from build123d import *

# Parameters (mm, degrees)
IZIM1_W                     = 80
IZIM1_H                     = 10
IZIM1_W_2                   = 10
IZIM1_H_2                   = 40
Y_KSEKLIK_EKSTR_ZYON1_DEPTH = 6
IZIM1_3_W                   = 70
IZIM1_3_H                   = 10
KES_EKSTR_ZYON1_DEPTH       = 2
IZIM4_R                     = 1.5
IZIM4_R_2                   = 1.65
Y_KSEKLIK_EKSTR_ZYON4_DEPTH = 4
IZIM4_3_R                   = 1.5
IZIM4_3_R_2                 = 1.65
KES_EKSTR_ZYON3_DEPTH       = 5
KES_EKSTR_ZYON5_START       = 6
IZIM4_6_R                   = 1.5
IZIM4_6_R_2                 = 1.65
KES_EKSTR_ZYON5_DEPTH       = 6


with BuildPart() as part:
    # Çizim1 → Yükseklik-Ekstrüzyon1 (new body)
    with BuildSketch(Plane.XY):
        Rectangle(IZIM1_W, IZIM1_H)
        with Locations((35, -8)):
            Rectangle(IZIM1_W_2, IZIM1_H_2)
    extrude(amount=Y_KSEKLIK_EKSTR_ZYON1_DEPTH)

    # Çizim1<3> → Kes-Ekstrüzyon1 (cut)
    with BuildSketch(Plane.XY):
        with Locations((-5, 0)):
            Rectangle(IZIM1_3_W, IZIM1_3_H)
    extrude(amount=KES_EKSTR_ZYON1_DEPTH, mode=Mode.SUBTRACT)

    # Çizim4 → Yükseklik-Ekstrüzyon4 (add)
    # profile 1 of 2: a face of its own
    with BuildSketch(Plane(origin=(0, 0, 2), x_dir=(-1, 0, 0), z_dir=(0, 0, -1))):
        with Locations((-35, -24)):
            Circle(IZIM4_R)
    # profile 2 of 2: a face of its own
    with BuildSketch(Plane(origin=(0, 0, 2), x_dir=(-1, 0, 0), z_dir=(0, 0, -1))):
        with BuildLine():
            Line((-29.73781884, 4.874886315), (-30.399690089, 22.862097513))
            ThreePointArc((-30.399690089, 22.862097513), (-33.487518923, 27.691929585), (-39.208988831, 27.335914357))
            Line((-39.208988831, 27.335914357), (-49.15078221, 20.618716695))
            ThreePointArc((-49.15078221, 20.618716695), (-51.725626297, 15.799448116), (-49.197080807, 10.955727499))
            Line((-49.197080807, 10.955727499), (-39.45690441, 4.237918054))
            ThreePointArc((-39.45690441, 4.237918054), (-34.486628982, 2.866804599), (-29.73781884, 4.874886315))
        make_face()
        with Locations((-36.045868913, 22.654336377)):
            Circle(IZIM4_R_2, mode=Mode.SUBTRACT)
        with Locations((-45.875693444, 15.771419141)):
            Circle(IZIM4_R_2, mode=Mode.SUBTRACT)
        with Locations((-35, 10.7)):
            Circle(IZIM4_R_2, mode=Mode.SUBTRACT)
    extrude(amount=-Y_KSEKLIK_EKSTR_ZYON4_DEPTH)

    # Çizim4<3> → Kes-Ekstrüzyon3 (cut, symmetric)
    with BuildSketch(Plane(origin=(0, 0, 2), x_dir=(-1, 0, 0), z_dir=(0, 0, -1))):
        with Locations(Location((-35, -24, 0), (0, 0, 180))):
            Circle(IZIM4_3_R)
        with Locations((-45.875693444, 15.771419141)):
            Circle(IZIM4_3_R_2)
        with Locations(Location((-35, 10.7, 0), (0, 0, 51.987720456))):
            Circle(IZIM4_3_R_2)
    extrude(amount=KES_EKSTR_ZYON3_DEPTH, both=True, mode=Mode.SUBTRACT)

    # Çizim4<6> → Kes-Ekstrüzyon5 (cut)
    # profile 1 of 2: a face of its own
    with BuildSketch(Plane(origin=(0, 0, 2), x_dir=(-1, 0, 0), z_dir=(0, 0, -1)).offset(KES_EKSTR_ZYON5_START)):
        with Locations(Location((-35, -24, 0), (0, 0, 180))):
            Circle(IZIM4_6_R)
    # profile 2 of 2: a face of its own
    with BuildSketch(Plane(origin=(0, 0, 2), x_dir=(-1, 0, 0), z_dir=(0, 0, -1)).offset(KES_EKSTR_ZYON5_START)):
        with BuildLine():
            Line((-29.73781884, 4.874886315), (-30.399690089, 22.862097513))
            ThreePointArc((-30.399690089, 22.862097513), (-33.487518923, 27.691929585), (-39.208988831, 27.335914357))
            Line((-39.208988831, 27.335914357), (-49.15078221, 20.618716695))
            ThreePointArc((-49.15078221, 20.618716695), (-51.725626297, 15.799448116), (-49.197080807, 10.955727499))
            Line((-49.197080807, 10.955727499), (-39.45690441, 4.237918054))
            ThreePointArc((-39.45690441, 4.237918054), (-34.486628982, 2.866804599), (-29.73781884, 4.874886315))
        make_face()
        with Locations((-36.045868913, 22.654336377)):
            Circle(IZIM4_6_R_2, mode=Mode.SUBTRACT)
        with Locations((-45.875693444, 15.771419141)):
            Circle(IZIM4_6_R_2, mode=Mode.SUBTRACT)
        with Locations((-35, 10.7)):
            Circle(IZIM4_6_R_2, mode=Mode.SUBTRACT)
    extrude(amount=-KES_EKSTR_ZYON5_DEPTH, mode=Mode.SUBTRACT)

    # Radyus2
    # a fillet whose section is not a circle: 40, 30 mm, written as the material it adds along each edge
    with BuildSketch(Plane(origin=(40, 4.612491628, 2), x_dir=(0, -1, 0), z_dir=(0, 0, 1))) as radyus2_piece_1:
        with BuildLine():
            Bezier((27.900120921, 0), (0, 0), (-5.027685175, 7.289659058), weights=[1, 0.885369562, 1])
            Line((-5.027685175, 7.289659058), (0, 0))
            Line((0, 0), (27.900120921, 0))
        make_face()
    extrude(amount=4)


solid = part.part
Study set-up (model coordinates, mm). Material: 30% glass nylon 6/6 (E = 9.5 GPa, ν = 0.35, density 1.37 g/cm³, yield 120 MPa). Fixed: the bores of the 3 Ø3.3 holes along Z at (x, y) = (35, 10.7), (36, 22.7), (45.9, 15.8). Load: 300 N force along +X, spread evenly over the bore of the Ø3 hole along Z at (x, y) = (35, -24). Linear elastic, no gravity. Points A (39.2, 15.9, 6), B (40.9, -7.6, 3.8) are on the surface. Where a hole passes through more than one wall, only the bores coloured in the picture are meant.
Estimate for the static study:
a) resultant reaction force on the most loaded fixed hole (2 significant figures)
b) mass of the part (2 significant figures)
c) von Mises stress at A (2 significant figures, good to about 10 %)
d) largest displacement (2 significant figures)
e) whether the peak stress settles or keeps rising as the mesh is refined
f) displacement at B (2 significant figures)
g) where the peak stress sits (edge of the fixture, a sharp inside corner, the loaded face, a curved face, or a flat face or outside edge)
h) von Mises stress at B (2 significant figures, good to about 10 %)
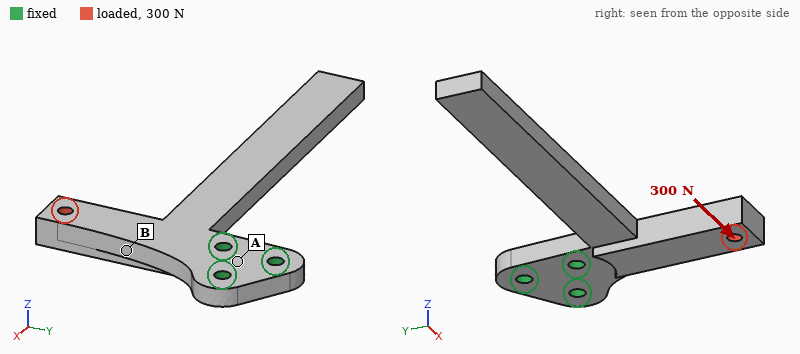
770 N
8.6 g
9.5 MPa
0.97 mm
keeps rising
0.23 mm
edge of the fixture
48 MPa
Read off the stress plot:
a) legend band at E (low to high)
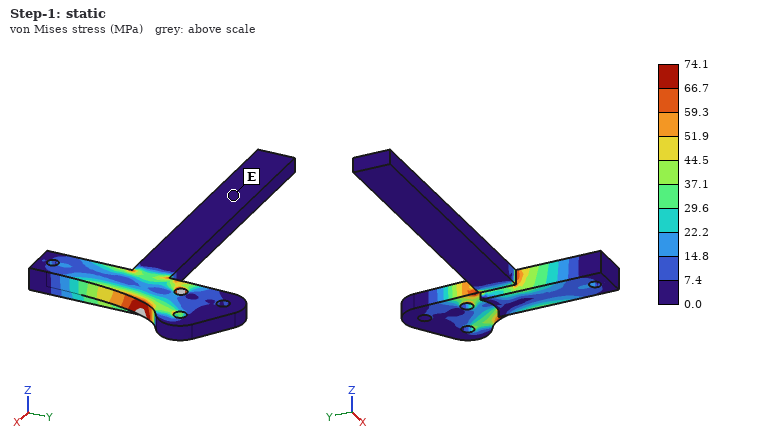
0.0 to 7.4 MPa
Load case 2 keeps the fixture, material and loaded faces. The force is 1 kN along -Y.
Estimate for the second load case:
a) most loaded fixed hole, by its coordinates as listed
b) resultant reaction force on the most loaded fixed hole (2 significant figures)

(35, 10.7)
830 N
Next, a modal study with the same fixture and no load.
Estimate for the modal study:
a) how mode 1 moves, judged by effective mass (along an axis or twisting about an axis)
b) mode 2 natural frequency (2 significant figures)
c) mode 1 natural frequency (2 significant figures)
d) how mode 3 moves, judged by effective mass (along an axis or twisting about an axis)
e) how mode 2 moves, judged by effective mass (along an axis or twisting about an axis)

along Z
710 Hz
290 Hz
along Z
along Y
